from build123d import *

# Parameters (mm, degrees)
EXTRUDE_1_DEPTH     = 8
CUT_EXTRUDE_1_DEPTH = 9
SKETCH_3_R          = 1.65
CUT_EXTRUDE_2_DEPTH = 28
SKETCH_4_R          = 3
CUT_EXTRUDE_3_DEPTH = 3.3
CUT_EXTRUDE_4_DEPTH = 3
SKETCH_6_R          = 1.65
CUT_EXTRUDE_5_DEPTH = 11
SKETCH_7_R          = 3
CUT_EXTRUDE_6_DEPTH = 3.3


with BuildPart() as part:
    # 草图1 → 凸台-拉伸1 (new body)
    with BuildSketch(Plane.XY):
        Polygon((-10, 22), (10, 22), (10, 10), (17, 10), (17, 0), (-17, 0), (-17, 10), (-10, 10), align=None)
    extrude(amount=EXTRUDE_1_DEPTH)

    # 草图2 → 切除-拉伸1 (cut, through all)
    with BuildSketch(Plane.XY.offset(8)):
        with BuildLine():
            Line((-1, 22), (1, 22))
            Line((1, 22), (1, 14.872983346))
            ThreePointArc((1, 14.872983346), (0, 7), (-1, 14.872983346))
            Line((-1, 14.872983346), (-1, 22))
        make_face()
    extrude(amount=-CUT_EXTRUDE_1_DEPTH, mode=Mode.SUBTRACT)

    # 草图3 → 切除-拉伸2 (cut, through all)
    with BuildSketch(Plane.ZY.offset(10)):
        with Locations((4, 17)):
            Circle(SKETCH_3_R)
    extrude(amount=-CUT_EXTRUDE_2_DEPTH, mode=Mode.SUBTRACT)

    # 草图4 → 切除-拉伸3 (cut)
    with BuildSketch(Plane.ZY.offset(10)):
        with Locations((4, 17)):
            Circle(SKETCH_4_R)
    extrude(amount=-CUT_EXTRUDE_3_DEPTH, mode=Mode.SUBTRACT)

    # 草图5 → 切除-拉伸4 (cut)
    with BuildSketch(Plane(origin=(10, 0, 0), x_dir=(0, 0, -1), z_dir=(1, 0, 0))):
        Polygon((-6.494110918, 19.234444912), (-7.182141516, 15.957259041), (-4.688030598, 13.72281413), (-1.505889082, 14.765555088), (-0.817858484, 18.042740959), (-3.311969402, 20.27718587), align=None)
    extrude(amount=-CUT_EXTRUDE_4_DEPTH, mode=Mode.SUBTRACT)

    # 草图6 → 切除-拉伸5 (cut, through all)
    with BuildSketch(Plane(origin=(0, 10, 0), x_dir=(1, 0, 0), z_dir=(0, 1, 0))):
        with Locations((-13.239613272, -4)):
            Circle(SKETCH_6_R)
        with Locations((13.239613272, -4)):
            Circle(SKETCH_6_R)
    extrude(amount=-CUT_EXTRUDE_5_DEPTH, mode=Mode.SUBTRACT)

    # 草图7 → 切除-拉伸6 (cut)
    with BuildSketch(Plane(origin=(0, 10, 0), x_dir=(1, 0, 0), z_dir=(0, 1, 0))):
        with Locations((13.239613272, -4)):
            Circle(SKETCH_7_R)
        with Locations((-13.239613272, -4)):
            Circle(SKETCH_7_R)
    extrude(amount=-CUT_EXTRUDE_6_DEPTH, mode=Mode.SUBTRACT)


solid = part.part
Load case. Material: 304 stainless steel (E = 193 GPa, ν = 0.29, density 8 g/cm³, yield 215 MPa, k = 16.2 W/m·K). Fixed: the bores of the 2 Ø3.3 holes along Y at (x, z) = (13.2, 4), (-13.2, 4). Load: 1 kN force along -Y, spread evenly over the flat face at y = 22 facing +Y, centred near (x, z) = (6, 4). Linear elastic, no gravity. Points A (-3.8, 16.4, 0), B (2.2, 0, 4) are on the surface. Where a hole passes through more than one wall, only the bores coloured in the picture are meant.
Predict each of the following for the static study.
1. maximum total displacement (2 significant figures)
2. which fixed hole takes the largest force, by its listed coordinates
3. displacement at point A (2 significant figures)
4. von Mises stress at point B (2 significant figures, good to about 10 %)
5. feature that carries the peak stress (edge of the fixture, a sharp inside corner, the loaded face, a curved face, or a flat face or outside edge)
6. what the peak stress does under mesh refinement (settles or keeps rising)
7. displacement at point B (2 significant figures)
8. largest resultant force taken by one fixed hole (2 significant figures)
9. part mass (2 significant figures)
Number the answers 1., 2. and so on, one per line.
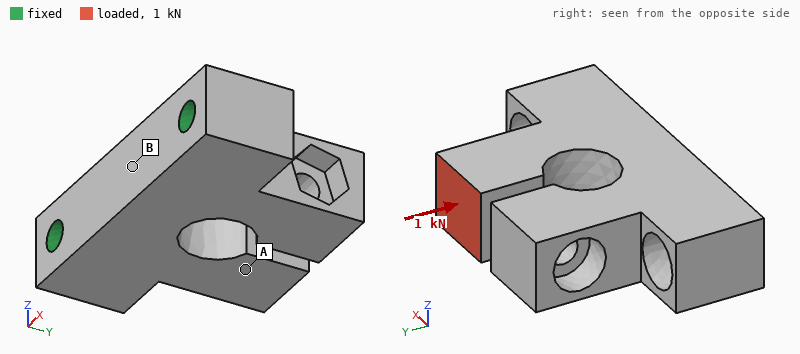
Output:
1. 9.2 µm
2. (13.2, 4)
3. 2.1 µm
4. 22 MPa
5. edge of the fixture
6. keeps rising
7. 1.9 µm
8. 760 N
9. 28 g
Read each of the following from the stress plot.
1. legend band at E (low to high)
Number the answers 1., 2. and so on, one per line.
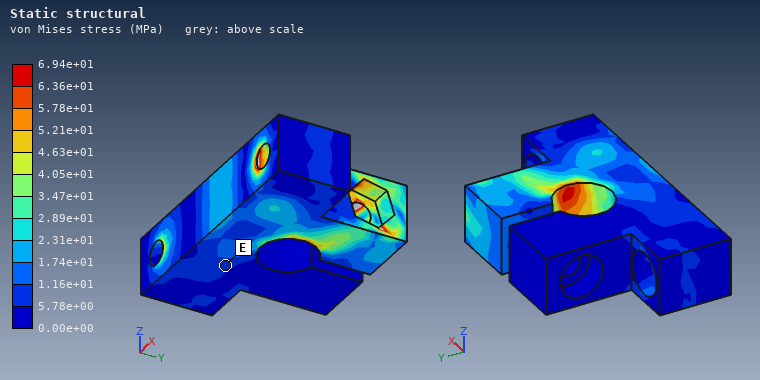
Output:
1. 5.78e+00 to 1.16e+01 MPa
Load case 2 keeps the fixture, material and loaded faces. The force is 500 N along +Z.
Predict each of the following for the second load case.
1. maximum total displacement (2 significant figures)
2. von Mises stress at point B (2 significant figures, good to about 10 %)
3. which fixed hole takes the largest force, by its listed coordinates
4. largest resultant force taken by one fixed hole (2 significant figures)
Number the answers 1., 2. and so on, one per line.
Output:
1. 34 µm
2. 18 MPa
3. (13.2, 4)
4. 420 N
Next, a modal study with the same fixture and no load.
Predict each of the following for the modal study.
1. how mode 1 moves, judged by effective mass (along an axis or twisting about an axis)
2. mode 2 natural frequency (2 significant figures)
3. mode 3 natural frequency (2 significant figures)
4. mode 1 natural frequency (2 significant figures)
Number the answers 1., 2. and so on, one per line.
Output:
1. along Z
2. 14 kHz
3. 14 kHz
4. 12 kHz
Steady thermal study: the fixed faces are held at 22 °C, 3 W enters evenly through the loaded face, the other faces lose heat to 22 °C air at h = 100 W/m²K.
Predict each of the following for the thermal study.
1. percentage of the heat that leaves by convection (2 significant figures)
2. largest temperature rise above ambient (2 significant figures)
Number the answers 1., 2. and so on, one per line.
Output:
1. 58 %
2. 48 K
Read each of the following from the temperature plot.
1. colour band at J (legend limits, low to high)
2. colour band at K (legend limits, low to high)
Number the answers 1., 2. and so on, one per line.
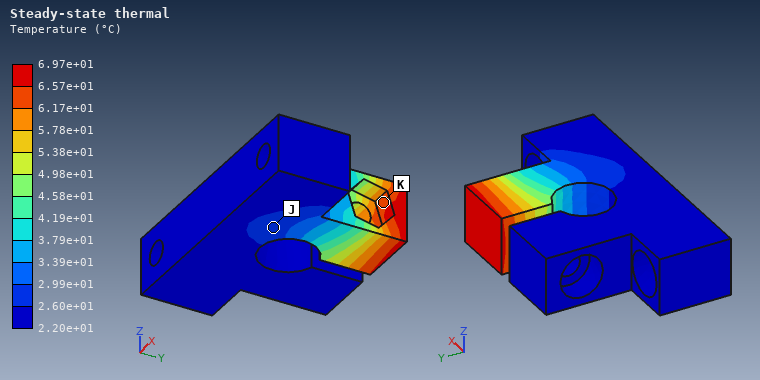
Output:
1. 2.60e+01 to 2.99e+01 °C
2. 6.17e+01 to 6.57e+01 °C
